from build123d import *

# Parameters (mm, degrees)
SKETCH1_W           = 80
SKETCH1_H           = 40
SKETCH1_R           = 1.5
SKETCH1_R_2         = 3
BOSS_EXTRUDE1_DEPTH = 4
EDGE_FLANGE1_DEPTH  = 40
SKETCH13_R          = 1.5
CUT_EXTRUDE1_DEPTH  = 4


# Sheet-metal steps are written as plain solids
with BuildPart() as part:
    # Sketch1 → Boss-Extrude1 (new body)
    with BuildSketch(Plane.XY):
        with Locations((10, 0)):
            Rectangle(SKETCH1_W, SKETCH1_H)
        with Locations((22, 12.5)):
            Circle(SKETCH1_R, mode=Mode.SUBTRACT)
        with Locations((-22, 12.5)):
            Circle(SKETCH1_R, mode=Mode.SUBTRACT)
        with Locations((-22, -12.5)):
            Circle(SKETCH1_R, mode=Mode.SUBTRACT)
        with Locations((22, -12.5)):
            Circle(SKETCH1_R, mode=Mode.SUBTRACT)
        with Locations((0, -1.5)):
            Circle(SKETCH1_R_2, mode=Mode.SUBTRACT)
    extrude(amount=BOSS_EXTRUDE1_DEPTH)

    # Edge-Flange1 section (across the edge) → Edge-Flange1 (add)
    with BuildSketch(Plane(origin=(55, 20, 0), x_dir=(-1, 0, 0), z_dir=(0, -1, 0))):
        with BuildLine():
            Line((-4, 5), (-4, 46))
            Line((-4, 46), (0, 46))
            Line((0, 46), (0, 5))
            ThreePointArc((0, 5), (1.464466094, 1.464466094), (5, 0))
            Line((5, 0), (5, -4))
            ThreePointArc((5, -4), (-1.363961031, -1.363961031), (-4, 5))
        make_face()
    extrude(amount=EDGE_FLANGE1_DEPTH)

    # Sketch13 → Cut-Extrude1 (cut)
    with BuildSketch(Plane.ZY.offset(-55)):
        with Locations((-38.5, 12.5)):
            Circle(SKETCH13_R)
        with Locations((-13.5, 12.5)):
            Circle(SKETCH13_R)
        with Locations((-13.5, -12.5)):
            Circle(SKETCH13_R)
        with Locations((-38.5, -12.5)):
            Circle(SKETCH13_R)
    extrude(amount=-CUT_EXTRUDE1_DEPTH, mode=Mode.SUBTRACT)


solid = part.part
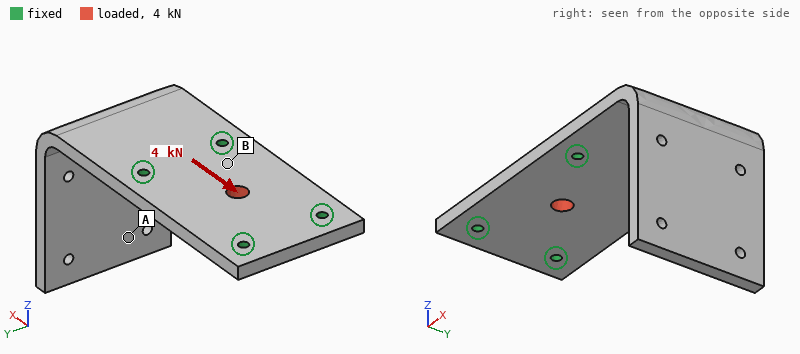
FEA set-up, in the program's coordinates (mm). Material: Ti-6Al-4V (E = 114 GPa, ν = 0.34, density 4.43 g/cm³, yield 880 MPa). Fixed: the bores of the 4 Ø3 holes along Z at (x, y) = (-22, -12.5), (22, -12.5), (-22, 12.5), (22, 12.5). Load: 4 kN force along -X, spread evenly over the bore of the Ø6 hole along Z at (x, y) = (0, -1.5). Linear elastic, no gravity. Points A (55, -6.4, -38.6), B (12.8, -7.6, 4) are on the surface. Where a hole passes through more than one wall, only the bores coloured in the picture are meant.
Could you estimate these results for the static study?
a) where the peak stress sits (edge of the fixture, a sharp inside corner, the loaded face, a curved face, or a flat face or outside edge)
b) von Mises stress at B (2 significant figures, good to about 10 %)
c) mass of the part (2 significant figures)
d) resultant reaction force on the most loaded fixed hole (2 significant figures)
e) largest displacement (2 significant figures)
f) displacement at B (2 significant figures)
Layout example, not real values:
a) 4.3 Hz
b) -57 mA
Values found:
a) the loaded face
b) 24 MPa
c) 92 g
d) 1.1 kN
e) 5.9 µm
f) 2.2 µm
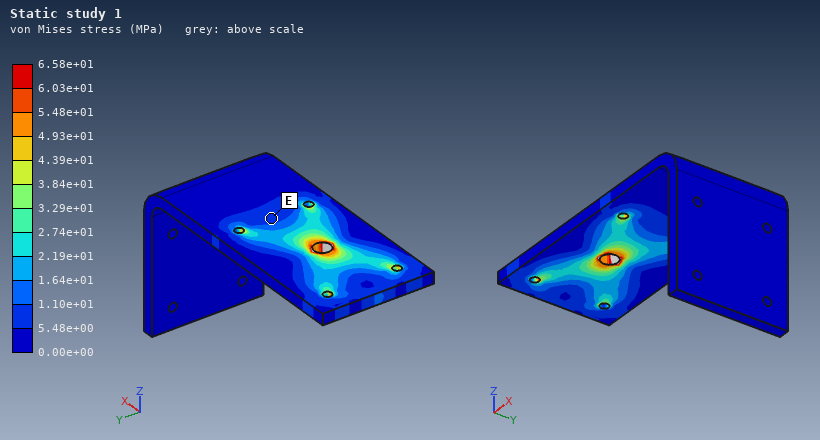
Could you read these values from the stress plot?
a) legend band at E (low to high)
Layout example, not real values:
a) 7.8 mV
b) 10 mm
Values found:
a) 5.48e+00 to 1.10e+01 MPa
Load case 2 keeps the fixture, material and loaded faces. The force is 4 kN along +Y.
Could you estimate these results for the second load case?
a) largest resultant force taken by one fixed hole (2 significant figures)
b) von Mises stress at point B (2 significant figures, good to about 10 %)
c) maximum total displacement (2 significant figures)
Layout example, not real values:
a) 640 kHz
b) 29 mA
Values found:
a) 1.2 kN
b) 29 MPa
c) 10 µm
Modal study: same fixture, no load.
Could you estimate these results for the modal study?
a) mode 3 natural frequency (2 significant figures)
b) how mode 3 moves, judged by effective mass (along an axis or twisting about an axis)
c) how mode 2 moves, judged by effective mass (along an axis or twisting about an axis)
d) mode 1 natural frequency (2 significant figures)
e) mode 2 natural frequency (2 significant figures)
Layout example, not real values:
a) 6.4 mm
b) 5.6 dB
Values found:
a) 1900 Hz
b) along Z
c) along Y
d) 650 Hz
e) 1100 Hz
